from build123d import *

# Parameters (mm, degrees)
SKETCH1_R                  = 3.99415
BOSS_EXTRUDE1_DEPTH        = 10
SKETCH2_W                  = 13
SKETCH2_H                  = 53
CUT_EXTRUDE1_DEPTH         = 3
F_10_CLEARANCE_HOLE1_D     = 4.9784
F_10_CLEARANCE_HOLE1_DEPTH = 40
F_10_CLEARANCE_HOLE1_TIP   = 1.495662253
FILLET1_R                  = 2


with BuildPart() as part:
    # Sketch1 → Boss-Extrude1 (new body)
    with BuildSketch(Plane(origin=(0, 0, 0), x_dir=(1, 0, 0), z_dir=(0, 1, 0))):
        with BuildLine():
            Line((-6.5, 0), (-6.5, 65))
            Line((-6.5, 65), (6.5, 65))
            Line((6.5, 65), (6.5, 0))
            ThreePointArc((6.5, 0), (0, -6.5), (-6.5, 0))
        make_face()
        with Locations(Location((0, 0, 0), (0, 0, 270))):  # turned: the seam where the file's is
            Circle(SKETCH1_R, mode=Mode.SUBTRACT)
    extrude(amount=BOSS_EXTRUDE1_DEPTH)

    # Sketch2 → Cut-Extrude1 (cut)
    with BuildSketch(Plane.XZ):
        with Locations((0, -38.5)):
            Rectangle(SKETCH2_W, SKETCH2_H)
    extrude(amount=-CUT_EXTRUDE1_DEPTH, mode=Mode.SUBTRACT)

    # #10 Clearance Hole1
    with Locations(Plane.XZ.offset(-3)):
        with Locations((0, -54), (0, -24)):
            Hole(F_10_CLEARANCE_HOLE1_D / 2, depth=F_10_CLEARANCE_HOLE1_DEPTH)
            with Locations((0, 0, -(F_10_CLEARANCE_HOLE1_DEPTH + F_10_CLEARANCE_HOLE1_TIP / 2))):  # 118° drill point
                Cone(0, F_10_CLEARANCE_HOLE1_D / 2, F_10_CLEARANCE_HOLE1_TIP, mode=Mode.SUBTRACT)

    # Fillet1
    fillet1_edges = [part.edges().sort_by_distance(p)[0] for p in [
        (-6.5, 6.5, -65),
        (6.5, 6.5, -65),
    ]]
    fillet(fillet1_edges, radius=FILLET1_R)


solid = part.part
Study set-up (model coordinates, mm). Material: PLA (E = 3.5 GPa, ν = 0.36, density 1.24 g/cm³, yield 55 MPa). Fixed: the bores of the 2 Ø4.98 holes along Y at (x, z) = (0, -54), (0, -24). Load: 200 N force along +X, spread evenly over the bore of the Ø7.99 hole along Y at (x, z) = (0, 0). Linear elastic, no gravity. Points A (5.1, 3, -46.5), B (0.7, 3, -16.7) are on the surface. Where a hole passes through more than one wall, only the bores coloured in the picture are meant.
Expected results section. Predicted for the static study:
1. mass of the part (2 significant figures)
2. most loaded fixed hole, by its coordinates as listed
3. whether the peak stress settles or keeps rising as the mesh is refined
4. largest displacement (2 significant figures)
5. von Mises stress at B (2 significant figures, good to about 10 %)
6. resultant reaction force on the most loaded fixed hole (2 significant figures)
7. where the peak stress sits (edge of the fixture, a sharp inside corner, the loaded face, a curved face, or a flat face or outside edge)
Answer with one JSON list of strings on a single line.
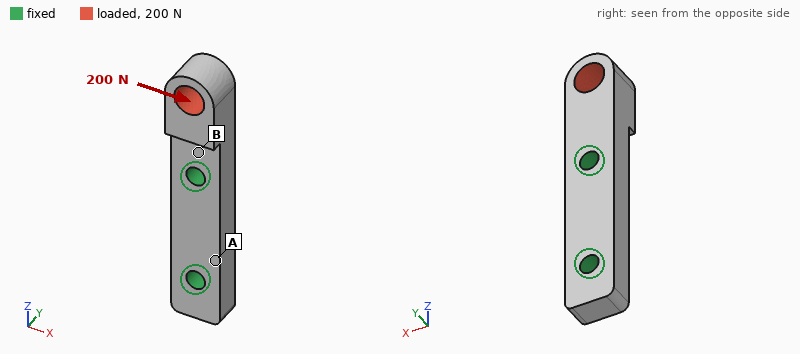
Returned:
["7.8 g", "(0, -24)", "keeps rising", "0.46 mm", "8.5 MPa", "260 N", "edge of the fixture"]
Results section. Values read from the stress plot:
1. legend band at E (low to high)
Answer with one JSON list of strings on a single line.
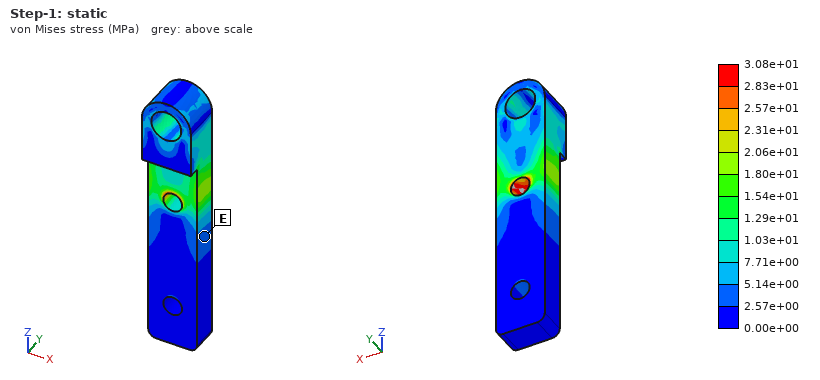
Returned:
["2.57e+00 to 5.14e+00 MPa"]
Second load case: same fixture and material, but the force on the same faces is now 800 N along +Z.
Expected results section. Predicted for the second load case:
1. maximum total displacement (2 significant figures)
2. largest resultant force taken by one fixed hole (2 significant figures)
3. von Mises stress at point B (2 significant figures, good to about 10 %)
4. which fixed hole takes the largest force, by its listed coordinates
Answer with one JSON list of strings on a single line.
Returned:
["0.33 mm", "770 N", "22 MPa", "(0, -24)"]
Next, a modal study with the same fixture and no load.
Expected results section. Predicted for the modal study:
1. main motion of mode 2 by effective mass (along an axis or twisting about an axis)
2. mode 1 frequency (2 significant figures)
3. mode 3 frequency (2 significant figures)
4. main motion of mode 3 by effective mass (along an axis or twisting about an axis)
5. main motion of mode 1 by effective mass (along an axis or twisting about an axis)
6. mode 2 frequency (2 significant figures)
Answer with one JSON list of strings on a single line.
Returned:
["along X", "2300 Hz", "6500 Hz", "twisting about Z", "along Y", "3100 Hz"]
